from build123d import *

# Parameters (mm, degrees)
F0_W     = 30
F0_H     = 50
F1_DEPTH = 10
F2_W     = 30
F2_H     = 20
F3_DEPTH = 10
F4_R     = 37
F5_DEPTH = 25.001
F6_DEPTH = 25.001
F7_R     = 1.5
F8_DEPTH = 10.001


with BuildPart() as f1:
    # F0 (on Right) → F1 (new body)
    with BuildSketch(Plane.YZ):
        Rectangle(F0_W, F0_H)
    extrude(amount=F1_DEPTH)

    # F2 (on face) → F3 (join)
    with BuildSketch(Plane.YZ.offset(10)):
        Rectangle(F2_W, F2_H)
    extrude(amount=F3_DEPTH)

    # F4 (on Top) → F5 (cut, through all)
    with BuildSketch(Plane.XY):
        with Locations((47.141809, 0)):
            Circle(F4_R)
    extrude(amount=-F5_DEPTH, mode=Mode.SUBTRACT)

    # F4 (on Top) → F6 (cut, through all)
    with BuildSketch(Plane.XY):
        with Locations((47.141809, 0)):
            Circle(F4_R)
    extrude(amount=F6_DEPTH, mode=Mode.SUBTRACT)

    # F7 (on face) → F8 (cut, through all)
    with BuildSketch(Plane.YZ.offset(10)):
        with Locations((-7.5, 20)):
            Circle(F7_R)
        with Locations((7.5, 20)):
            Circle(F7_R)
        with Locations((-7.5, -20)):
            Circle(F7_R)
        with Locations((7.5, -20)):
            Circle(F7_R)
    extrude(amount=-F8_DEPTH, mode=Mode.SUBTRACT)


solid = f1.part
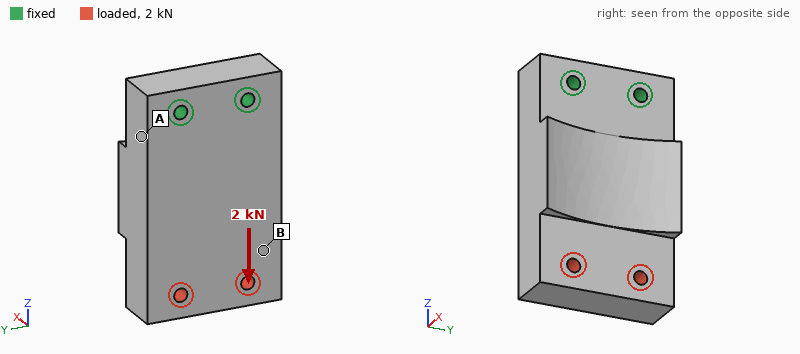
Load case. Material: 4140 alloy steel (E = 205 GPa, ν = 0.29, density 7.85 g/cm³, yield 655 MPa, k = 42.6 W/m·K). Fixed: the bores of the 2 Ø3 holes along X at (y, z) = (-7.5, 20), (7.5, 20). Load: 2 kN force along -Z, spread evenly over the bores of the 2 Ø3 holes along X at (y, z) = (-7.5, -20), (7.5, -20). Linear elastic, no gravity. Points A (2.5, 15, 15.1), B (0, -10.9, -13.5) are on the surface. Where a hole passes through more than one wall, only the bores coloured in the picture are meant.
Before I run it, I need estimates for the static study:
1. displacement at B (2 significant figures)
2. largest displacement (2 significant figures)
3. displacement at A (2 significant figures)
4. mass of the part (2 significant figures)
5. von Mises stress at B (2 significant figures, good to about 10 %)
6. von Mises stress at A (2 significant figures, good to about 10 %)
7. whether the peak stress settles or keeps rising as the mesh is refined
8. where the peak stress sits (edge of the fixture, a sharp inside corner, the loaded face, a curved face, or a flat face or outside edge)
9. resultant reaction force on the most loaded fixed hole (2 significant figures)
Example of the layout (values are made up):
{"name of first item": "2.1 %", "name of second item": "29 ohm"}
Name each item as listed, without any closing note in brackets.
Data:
{"displacement at B": "1.4 µm", "largest displacement": "1.9 µm", "displacement at A": "0.39 µm", "mass of the part": "120 g", "von Mises stress at B": "7.3 MPa", "von Mises stress at A": "3.0 MPa", "whether the peak stress settles or keeps rising as the mesh is refined": "keeps rising", "where the peak stress sits": "edge of the fixture", "resultant reaction force on the most loaded fixed hole": "1.0 kN"}
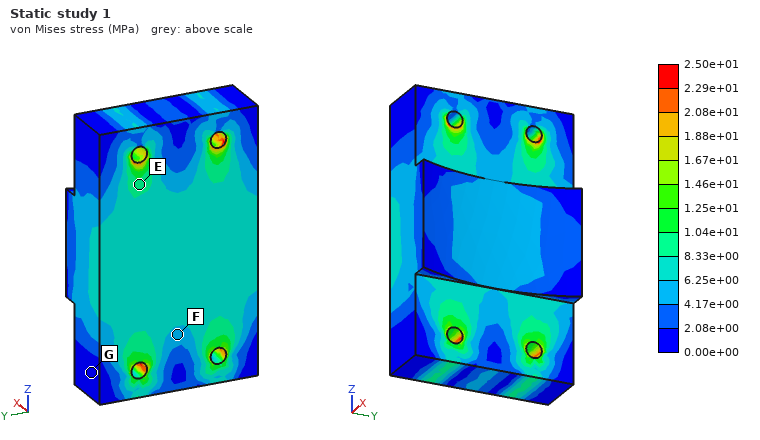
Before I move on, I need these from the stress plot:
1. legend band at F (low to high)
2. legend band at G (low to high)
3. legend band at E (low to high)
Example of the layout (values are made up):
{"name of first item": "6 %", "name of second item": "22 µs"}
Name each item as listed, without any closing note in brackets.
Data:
{"legend band at F": "4.17e+00 to 6.25e+00 MPa", "legend band at G": "0.00e+00 to 2.08e+00 MPa", "legend band at E": "8.33e+00 to 1.04e+01 MPa"}
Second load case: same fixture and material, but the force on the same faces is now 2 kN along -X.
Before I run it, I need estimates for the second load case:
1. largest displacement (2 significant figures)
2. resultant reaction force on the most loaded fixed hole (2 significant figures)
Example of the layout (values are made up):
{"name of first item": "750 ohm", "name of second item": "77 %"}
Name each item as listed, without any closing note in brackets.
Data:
{"largest displacement": "0.11 mm", "resultant reaction force on the most loaded fixed hole": "1.0 kN"}
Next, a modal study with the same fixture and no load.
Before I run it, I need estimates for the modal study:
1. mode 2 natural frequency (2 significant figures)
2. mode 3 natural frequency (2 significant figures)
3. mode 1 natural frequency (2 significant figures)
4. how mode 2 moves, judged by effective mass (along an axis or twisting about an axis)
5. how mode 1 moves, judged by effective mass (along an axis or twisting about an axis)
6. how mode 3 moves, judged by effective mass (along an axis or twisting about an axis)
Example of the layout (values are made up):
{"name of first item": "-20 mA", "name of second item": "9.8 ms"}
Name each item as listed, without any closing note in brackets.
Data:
{"mode 2 natural frequency": "8000 Hz", "mode 3 natural frequency": "11 kHz", "mode 1 natural frequency": "3800 Hz", "how mode 2 moves, judged by effective mass": "along Y", "how mode 1 moves, judged by effective mass": "along X", "how mode 3 moves, judged by effective mass": "twisting about Z"}
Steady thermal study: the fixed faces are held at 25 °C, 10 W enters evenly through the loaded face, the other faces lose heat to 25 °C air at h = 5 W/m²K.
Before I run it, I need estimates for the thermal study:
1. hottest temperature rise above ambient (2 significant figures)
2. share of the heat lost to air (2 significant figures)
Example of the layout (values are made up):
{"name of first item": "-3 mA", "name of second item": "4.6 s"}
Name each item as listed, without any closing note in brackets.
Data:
{"hottest temperature rise above ambient": "32 K", "share of the heat lost to air": "3.6 %"}
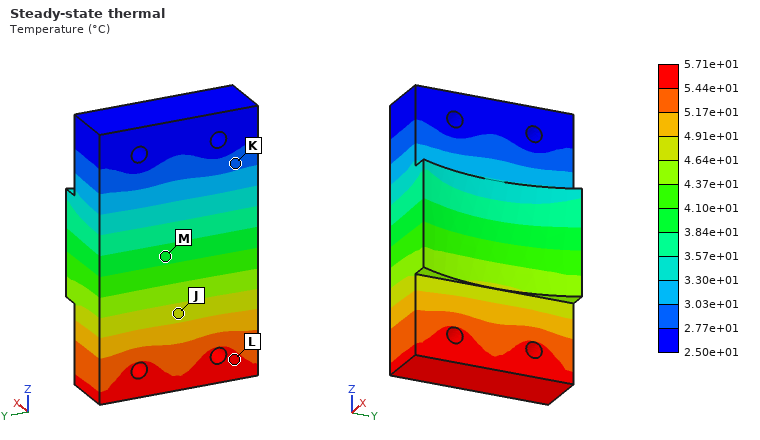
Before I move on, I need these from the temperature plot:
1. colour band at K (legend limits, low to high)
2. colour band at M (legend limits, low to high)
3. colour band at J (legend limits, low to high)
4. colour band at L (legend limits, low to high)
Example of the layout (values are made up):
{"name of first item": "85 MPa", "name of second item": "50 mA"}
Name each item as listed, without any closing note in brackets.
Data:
{"colour band at K": "2.77e+01 to 3.03e+01 °C", "colour band at M": "3.84e+01 to 4.10e+01 °C", "colour band at J": "4.64e+01 to 4.91e+01 °C", "colour band at L": "5.44e+01 to 5.71e+01 °C"}
